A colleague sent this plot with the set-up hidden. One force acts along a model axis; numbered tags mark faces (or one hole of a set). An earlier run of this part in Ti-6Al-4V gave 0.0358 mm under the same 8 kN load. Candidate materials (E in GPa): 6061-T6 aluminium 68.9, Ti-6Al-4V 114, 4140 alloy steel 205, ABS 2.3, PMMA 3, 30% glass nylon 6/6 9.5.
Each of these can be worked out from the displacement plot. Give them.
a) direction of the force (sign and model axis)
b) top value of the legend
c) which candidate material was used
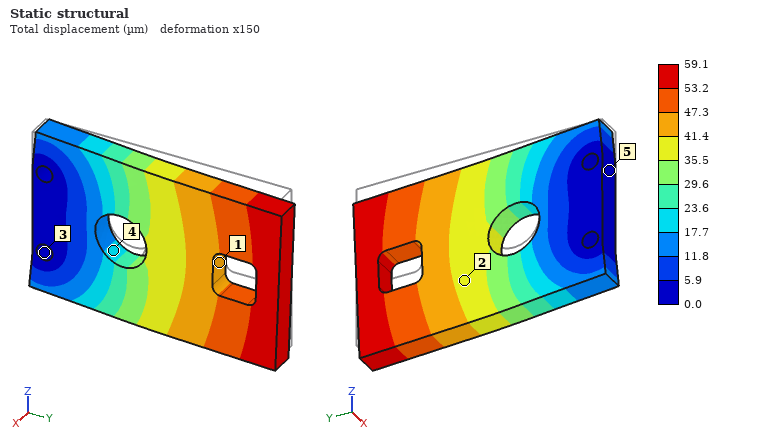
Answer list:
-Z
59.1 µm
6061-T6 aluminium
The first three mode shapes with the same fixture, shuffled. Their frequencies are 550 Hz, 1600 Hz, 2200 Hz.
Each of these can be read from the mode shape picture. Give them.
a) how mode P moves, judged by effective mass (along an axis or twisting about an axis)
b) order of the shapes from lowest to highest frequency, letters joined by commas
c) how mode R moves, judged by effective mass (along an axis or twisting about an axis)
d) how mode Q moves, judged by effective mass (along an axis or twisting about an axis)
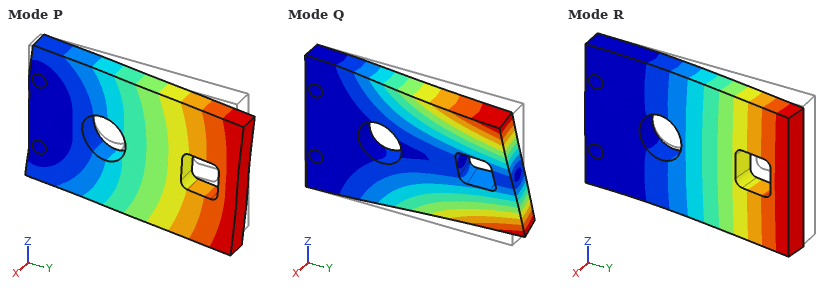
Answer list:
along Z
R, Q, P
along X
twisting about Y
